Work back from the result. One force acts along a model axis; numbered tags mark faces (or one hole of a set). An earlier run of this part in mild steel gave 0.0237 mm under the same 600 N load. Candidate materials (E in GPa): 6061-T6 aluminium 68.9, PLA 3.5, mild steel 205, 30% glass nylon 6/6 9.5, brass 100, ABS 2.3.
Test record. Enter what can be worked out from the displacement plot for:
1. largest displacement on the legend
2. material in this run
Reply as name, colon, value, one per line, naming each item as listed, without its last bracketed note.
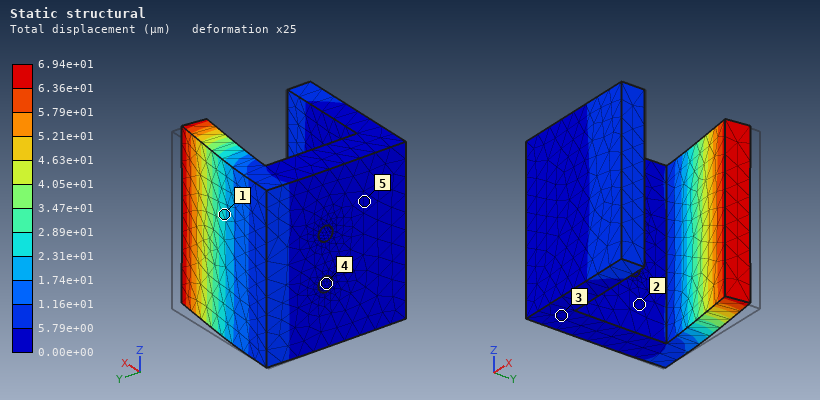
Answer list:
largest displacement on the legend: 6.94e+01 µm
material in this run: 6061-T6 aluminium
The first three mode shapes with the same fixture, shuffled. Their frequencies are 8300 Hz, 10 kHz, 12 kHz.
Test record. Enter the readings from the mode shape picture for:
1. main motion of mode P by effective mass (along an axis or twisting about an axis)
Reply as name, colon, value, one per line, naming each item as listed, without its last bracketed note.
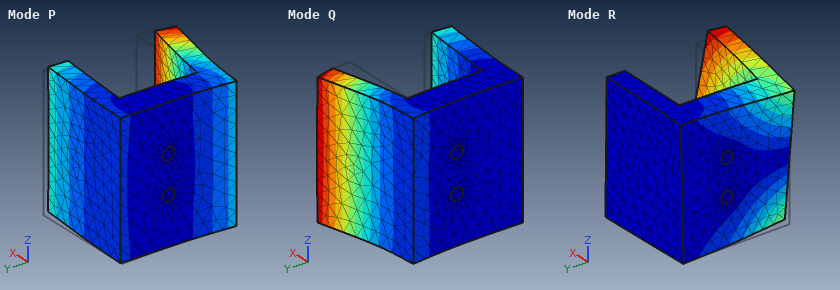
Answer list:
main motion of mode P by effective mass: along Y
